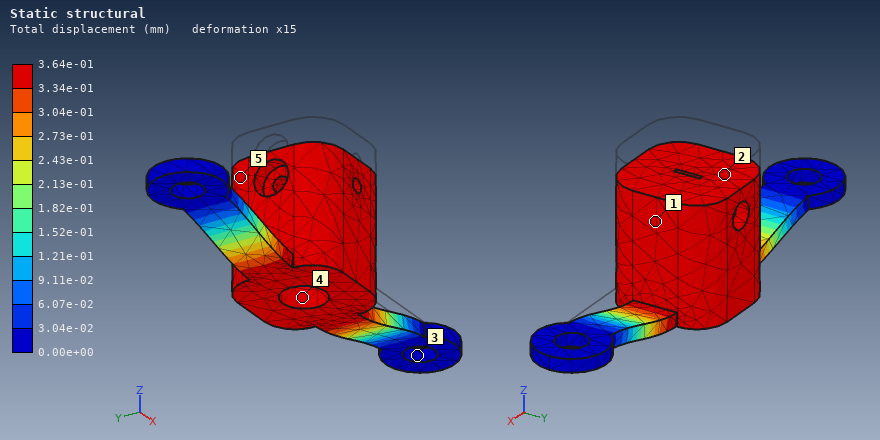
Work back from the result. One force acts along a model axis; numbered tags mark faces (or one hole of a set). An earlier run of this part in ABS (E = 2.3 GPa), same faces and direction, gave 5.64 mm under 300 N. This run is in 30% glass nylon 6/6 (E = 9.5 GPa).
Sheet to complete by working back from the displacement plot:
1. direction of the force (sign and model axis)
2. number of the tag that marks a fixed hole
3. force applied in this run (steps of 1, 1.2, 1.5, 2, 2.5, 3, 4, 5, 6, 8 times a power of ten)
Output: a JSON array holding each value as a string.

["-Z", "3", "80 N"]
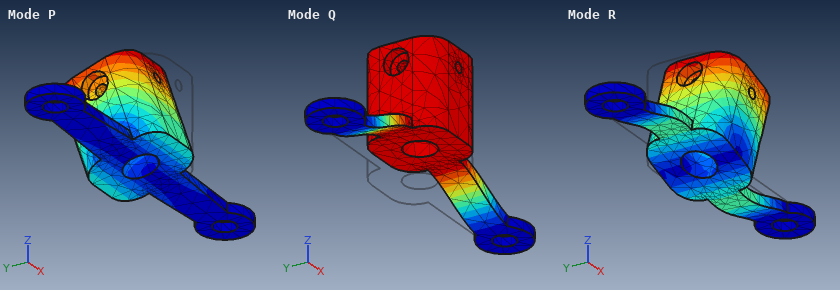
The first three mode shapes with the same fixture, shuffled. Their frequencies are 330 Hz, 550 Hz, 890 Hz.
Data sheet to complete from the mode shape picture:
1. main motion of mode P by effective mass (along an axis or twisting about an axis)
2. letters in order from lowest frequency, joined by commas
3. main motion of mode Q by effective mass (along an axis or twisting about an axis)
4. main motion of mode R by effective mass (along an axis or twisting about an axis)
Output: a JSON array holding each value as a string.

["along Y", "P, Q, R", "along Z", "along X"]
